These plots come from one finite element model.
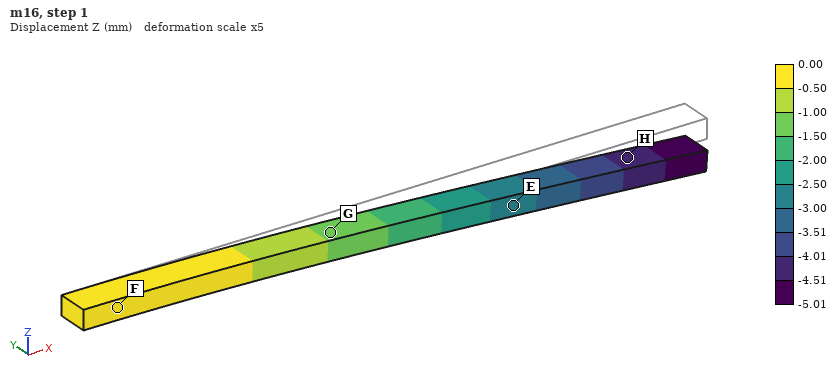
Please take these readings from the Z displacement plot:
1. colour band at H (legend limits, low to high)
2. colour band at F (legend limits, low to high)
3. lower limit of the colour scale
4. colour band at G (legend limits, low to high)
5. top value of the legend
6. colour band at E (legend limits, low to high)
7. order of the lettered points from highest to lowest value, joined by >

-4.51 to -4.01 mm
-0.50 to 0.00 mm
-5.01 mm
-1.50 to -1.00 mm
0.00 mm
-3.00 to -2.50 mm
F > G > E > H
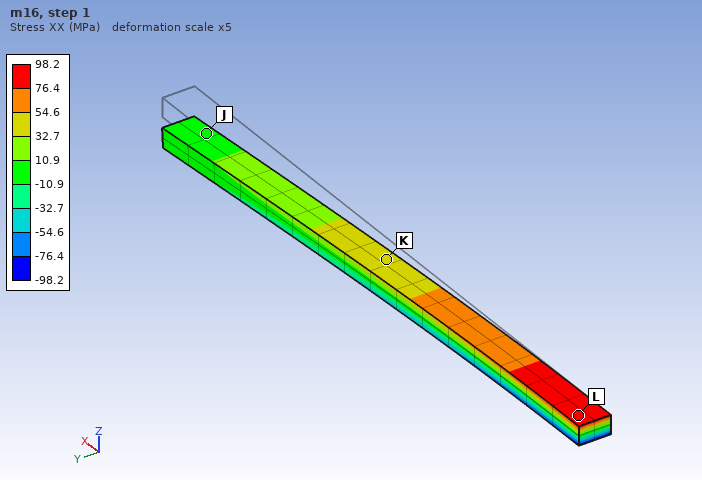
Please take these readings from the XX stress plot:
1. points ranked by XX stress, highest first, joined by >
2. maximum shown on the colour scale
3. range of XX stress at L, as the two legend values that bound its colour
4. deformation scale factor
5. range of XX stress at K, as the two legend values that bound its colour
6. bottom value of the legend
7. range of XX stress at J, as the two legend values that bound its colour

L > K > J
98.2 MPa
76.4 to 98.2 MPa
5
32.7 to 54.6 MPa
-98.2 MPa
-10.9 to 10.9 MPa
